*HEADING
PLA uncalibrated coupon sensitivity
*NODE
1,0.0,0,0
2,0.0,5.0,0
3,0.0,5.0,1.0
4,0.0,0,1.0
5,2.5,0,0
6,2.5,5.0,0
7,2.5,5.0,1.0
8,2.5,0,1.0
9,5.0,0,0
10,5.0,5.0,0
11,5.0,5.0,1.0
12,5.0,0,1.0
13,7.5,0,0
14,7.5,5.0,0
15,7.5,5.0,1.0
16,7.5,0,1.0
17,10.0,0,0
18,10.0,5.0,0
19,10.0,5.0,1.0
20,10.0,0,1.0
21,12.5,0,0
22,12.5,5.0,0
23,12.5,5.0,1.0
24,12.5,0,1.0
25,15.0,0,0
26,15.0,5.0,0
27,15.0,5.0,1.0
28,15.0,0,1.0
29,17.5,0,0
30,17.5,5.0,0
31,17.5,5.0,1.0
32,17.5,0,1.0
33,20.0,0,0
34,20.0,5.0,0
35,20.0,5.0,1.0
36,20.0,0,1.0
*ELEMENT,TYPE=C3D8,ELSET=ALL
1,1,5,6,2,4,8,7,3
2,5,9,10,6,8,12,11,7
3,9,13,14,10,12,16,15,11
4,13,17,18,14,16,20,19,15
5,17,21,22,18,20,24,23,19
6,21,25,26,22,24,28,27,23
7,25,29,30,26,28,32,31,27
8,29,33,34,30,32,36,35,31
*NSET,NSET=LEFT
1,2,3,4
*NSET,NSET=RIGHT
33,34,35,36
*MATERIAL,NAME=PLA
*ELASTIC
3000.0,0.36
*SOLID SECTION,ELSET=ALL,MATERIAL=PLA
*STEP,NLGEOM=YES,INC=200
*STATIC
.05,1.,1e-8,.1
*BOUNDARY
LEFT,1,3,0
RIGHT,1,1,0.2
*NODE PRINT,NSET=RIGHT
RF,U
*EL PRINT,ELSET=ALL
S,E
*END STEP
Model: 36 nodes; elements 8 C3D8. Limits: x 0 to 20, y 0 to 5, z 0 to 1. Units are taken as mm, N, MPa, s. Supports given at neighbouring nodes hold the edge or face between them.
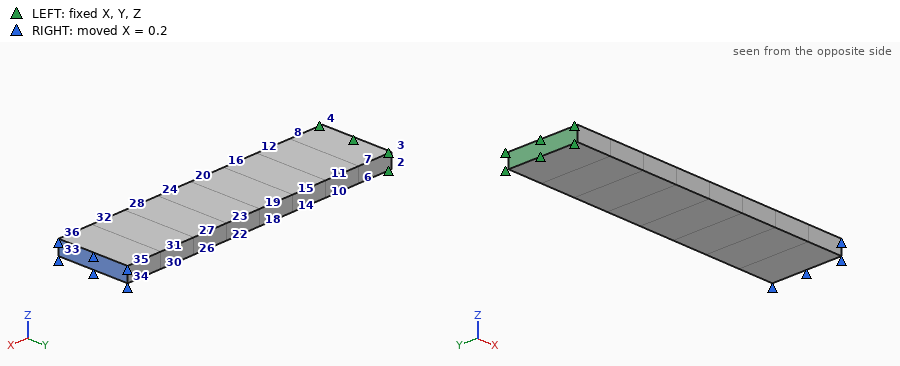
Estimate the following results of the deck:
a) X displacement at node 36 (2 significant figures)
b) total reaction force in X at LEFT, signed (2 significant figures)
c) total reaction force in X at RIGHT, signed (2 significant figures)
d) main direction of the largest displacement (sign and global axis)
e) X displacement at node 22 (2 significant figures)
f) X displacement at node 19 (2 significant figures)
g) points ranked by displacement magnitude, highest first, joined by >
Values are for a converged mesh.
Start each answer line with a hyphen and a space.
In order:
- 0.20 mm
- -150 N
- 150 N
- +X
- 0.12 mm
- 0.099 mm
- node 36 > node 31 > node 22 > node 19 > node 3
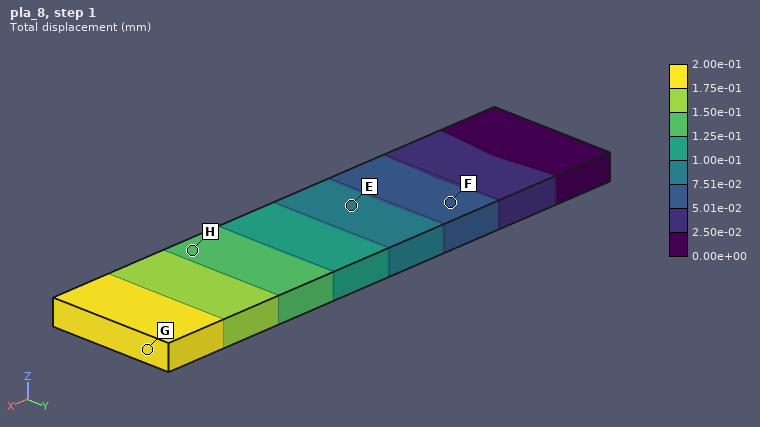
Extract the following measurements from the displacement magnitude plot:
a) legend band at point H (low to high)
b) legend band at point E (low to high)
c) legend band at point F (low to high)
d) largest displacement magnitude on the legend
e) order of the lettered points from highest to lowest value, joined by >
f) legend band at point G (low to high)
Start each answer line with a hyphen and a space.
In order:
- 1.25e-01 to 1.50e-01 mm
- 7.51e-02 to 1.00e-01 mm
- 5.01e-02 to 7.51e-02 mm
- 2.00e-01 mm
- G > H > E > F
- 1.75e-01 to 2.00e-01 mm
